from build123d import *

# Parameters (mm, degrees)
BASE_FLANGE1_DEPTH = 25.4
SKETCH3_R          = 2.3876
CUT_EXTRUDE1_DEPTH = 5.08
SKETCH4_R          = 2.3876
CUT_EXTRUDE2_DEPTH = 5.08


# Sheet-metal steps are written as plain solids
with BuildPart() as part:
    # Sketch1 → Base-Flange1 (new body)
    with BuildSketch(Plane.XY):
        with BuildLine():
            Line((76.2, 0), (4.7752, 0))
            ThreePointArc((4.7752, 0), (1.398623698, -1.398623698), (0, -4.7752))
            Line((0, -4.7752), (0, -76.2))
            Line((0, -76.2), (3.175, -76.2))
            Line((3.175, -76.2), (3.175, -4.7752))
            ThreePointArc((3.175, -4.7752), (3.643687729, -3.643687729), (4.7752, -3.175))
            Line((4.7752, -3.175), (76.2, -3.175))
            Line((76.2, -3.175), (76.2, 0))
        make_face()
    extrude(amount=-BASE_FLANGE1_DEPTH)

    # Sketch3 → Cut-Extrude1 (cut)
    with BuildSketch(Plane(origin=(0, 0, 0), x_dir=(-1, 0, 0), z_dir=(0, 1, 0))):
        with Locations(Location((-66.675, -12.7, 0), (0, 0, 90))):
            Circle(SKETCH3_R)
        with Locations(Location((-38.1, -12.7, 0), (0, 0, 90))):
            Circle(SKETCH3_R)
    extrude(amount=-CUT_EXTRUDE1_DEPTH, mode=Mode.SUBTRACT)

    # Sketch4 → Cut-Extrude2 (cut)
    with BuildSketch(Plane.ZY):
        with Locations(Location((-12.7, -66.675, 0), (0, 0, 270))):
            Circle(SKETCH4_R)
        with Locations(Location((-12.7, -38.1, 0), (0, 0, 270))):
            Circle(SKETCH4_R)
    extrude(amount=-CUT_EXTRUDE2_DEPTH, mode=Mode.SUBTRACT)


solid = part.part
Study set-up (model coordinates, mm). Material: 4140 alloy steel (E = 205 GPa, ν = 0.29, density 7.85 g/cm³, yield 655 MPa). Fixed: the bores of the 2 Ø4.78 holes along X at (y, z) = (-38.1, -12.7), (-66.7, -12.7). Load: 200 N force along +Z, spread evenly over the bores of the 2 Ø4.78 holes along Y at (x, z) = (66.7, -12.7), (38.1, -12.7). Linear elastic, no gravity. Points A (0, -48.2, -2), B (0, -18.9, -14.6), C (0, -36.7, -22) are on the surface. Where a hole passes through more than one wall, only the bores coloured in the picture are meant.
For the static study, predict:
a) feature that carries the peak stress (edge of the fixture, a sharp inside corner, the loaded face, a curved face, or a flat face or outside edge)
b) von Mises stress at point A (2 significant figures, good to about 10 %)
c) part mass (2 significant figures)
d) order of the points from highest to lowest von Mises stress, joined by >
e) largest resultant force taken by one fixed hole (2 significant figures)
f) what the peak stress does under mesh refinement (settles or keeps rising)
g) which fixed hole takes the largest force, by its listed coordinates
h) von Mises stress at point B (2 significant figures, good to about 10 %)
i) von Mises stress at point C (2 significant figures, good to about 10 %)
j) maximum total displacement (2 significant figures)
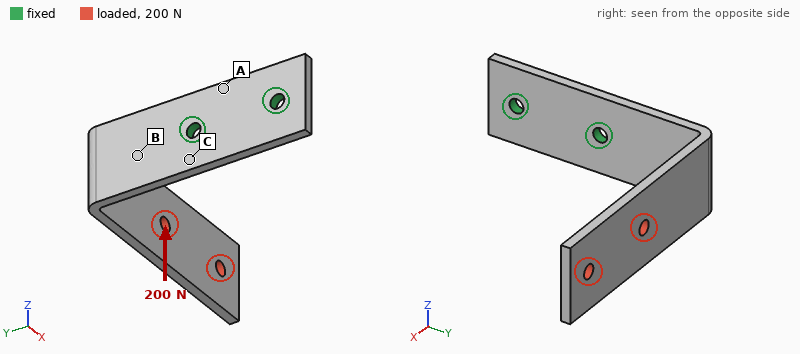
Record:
edge of the fixture
48 MPa
92 g
B > C > A
390 N
keeps rising
(-38.1, -12.7)
210 MPa
150 MPa
1.3 mm
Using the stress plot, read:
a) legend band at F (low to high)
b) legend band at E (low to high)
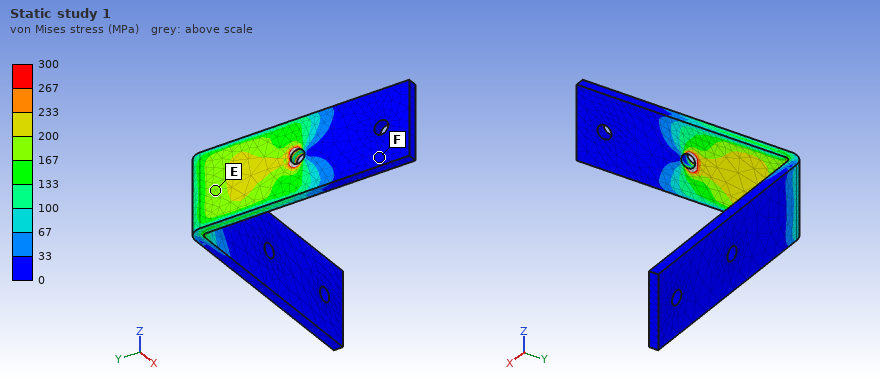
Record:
0 to 33 MPa
167 to 200 MPa
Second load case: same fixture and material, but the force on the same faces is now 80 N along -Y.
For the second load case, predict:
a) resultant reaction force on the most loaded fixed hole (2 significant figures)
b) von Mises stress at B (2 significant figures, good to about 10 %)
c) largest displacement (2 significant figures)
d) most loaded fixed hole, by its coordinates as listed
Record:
71 N
86 MPa
1.2 mm
(-38.1, -12.7)
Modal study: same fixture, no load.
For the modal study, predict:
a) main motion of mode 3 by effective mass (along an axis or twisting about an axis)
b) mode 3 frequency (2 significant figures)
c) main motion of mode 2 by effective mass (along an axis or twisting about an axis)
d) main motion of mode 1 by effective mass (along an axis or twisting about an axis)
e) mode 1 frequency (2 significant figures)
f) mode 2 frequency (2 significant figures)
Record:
along X
960 Hz
along Z
along Y
270 Hz
420 Hz
